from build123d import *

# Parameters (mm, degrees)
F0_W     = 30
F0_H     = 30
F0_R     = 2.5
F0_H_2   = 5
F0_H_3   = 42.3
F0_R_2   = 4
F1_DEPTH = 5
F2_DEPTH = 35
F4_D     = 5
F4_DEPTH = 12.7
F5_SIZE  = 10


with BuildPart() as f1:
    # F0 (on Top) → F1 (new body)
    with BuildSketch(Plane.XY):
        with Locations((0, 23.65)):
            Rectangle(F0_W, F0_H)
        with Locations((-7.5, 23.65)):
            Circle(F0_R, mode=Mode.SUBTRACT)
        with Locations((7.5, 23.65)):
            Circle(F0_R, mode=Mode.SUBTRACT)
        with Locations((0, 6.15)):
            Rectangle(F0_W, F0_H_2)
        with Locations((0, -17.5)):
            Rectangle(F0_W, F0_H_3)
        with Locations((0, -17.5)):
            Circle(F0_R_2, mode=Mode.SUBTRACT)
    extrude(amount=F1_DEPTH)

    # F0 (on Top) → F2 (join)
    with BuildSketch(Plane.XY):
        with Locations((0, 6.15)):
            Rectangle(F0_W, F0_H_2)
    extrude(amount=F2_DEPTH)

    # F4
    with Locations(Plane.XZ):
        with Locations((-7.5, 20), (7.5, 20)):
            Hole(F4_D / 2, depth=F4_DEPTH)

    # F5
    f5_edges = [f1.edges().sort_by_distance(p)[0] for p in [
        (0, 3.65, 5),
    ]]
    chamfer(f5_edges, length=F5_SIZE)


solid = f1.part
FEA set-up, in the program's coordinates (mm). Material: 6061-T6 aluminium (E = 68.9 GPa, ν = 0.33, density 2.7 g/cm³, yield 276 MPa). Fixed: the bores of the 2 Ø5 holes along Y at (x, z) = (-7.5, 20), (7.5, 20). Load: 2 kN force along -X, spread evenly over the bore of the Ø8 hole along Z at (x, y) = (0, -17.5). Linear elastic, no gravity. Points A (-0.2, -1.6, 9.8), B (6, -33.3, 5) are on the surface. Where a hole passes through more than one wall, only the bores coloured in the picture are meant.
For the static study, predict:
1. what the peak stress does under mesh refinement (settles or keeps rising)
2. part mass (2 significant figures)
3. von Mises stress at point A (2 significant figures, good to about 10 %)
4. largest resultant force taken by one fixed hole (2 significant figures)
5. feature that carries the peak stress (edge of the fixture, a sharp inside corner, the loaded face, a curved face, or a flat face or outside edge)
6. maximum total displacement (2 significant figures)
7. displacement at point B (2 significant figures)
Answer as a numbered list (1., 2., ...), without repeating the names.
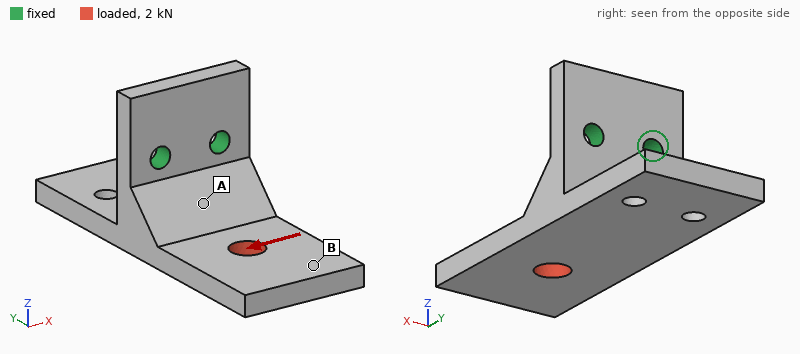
1. keeps rising
2. 46 g
3. 88 MPa
4. 3.2 kN
5. edge of the fixture
6. 0.21 mm
7. 0.18 mm
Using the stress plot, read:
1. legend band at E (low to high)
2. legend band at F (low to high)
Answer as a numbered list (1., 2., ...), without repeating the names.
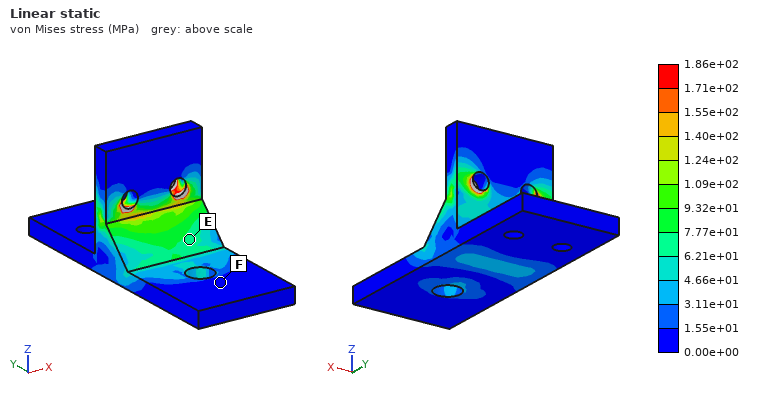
1. 6.21e+01 to 7.77e+01 MPa
2. 0.00e+00 to 1.55e+01 MPa
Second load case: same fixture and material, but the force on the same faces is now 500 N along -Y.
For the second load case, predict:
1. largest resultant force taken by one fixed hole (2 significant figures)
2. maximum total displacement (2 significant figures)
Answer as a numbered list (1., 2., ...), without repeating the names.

1. 250 N
2. 0.10 mm
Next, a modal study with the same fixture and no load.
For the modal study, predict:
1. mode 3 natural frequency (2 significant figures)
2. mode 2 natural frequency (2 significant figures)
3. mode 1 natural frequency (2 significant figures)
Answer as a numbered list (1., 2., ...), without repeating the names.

1. 3700 Hz
2. 3600 Hz
3. 1700 Hz
